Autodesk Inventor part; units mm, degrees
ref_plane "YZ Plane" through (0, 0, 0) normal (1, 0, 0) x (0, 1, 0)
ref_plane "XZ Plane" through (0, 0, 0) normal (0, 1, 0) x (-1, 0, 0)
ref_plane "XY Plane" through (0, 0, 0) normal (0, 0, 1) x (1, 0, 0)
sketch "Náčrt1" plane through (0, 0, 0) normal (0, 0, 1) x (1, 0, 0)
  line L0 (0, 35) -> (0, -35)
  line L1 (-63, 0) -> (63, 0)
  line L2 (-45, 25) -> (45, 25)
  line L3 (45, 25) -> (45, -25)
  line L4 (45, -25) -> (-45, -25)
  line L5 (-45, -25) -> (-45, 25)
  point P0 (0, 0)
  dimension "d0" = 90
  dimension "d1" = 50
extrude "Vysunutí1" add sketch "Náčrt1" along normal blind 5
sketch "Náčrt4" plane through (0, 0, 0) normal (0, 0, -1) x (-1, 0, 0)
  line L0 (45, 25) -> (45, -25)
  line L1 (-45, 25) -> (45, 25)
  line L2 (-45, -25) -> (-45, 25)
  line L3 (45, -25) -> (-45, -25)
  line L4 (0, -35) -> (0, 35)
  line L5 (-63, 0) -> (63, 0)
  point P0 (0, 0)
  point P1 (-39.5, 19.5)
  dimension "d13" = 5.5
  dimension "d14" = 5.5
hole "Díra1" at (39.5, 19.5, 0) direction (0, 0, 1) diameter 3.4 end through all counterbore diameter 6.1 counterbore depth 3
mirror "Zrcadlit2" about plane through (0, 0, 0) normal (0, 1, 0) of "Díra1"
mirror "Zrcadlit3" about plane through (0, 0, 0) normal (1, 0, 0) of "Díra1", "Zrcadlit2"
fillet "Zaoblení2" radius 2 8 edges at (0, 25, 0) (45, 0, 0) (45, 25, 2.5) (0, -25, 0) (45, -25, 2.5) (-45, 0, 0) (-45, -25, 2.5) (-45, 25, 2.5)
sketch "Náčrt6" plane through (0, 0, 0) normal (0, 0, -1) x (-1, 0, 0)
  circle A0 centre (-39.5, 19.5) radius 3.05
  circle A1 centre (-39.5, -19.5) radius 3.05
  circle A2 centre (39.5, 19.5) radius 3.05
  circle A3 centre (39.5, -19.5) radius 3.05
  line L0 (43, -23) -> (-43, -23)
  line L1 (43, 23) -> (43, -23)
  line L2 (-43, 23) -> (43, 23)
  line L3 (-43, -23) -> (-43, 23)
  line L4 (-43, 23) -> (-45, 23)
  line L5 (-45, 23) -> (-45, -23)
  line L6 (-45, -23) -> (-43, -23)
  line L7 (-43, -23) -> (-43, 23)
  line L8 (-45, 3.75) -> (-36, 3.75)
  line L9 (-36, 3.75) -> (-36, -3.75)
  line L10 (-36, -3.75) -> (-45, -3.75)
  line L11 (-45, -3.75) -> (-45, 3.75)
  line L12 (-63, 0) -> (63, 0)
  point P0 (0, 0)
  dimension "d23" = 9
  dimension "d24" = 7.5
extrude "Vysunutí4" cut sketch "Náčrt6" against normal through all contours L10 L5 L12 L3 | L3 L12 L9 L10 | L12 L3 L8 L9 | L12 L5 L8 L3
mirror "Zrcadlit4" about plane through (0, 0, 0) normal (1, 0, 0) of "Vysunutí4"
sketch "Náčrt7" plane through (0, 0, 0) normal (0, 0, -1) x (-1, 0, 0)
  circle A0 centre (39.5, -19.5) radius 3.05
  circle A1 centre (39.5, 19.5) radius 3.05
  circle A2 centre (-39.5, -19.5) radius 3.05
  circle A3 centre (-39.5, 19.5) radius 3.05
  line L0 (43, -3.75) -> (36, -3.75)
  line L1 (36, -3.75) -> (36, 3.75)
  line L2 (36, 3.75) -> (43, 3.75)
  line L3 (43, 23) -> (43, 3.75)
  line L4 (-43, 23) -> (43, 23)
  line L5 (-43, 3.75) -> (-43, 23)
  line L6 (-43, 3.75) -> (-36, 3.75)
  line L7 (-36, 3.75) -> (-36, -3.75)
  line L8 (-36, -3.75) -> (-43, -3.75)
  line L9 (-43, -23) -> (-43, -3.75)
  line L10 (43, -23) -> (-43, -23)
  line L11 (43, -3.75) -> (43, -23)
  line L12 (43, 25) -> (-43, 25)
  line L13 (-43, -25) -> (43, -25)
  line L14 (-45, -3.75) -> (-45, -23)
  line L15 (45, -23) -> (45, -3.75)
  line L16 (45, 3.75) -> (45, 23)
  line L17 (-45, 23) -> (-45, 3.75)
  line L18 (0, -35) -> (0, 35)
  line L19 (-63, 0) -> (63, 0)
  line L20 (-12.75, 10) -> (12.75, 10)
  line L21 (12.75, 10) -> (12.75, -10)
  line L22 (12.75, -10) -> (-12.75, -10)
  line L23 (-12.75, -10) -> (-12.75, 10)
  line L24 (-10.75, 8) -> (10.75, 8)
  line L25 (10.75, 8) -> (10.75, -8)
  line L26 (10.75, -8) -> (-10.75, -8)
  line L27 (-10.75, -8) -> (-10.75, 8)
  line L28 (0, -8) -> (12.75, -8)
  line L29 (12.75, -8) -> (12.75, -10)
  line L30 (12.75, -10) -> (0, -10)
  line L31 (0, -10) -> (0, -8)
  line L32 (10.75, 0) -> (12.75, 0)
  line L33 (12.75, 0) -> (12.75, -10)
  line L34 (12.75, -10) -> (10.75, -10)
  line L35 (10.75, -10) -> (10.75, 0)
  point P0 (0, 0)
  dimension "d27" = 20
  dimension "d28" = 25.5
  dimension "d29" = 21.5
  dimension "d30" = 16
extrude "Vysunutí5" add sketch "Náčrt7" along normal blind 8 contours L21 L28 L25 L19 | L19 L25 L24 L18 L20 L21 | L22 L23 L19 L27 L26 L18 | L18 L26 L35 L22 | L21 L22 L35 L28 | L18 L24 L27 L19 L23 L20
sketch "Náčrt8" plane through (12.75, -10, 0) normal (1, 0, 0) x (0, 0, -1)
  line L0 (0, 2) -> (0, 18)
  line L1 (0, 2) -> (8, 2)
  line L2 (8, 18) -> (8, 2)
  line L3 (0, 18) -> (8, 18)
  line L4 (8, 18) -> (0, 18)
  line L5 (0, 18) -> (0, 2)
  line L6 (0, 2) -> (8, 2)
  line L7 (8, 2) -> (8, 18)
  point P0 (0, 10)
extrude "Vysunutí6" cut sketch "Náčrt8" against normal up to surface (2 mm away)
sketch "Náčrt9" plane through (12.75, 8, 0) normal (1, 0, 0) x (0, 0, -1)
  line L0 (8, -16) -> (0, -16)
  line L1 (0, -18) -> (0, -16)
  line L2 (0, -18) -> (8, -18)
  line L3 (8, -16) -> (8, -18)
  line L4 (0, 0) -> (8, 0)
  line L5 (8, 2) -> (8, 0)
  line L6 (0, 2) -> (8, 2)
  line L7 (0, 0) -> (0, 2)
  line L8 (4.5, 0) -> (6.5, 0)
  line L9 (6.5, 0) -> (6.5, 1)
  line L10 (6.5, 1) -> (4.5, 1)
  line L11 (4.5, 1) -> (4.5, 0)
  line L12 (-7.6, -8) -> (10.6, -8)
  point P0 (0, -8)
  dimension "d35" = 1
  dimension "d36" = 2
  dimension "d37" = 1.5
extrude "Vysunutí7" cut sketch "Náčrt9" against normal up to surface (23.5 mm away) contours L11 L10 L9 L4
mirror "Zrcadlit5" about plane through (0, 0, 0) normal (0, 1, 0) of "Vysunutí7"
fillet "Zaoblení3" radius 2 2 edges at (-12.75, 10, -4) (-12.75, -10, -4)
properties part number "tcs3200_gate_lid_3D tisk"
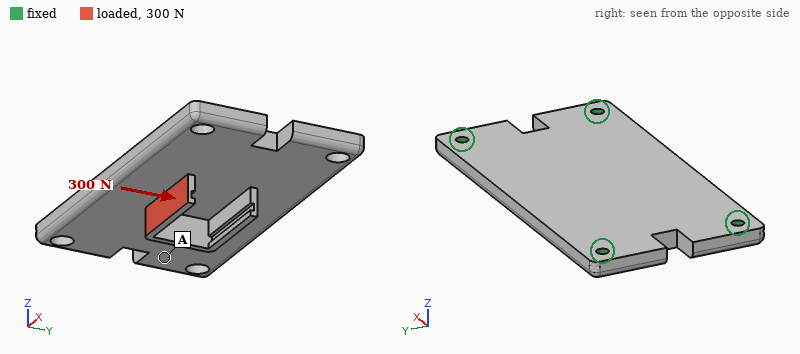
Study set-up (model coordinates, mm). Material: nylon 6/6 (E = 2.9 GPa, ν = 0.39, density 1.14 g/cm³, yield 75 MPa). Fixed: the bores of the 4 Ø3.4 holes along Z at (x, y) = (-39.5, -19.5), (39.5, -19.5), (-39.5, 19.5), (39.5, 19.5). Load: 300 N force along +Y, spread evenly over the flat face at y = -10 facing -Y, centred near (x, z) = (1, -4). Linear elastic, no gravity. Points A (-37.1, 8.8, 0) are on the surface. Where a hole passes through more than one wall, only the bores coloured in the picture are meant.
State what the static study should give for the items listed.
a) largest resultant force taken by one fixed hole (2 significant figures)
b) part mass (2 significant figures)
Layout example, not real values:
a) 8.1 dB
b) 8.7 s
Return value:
a) 120 N
b) 25 g
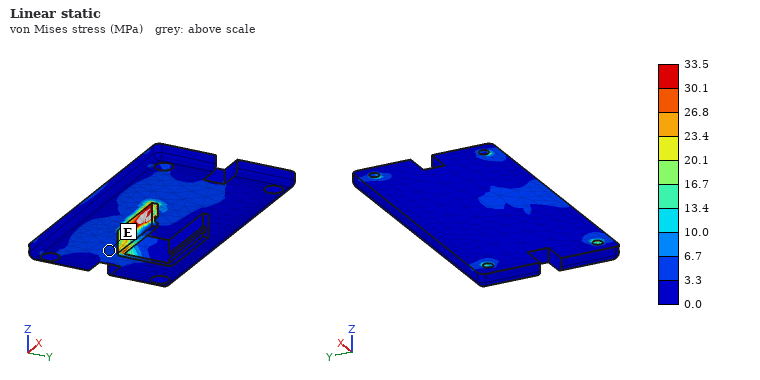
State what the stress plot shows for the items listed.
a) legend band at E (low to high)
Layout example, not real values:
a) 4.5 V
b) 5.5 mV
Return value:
a) 3.3 to 6.7 MPa
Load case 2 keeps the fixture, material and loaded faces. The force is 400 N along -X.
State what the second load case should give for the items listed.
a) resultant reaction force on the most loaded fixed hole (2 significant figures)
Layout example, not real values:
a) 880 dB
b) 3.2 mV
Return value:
a) 130 N
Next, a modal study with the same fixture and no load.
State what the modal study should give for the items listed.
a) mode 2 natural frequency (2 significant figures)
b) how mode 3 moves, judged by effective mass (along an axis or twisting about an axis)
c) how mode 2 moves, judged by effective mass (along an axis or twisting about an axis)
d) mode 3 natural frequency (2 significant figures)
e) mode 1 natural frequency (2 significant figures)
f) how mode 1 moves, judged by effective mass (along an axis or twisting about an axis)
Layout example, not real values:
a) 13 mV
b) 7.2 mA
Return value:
a) 1500 Hz
b) twisting about Y
c) twisting about X
d) 2400 Hz
e) 950 Hz
f) along Z
